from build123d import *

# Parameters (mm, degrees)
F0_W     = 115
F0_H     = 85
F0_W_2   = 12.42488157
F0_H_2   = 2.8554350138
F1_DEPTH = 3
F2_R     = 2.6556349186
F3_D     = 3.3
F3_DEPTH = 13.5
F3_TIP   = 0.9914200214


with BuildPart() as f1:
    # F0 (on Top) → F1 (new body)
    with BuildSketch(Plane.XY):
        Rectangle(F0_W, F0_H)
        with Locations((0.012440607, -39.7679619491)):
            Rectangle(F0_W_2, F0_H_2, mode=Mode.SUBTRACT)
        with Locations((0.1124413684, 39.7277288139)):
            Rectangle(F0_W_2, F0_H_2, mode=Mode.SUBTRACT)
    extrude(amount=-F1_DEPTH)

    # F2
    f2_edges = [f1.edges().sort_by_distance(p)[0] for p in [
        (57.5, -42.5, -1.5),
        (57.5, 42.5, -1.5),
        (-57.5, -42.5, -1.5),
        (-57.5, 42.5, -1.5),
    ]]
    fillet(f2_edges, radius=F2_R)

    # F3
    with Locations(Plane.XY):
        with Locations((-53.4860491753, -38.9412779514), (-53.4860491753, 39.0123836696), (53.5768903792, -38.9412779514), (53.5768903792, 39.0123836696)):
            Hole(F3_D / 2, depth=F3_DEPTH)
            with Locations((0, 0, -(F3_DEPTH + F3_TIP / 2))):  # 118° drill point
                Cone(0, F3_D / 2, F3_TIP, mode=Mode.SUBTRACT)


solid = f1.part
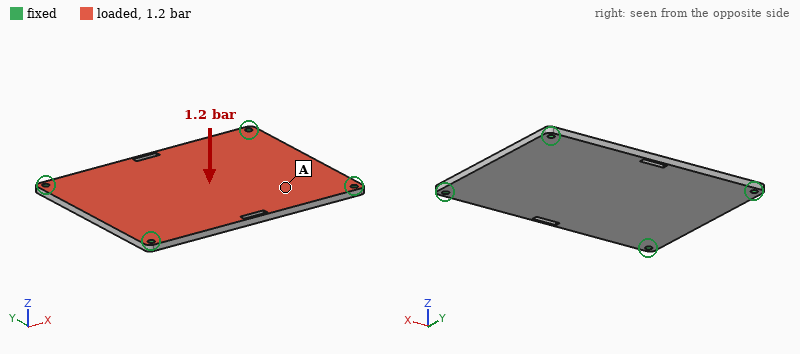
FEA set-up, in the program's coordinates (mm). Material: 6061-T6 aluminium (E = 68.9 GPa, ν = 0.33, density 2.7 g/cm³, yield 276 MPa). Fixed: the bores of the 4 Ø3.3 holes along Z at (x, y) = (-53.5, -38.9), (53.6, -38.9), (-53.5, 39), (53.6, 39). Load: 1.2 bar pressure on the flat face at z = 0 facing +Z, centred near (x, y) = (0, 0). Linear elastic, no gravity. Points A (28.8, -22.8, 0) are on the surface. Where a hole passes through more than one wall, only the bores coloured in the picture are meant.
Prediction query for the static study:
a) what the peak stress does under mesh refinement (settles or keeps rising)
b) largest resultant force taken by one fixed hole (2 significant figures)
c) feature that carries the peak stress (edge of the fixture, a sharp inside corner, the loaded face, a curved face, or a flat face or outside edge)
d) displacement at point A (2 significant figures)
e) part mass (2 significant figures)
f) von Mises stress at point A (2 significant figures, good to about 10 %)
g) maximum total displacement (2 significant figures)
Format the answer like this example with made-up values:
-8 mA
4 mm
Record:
keeps rising
290 N
edge of the fixture
0.32 mm
78 g
25 MPa
0.53 mm
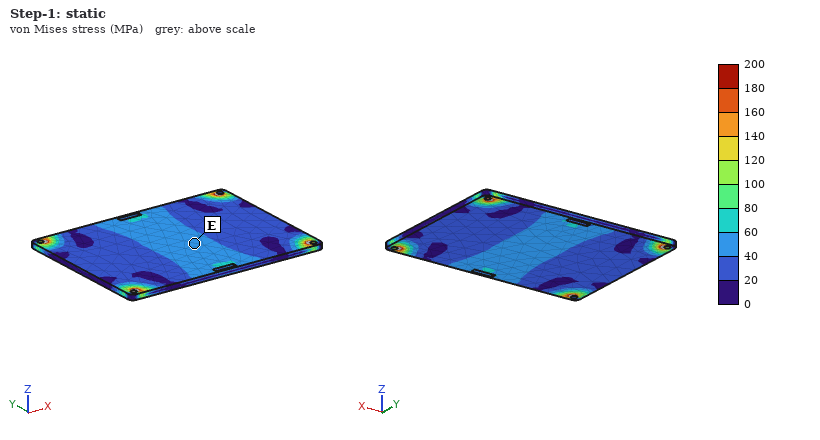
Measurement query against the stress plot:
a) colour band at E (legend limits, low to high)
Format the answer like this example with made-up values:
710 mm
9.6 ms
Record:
40 to 60 MPa
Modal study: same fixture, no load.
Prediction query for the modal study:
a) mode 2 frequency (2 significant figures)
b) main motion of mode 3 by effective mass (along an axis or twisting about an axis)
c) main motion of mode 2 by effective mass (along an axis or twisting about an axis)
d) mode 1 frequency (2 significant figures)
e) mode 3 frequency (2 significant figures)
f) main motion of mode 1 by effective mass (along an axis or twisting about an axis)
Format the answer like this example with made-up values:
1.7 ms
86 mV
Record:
1700 Hz
twisting about Y
twisting about X
980 Hz
2300 Hz
along Z
